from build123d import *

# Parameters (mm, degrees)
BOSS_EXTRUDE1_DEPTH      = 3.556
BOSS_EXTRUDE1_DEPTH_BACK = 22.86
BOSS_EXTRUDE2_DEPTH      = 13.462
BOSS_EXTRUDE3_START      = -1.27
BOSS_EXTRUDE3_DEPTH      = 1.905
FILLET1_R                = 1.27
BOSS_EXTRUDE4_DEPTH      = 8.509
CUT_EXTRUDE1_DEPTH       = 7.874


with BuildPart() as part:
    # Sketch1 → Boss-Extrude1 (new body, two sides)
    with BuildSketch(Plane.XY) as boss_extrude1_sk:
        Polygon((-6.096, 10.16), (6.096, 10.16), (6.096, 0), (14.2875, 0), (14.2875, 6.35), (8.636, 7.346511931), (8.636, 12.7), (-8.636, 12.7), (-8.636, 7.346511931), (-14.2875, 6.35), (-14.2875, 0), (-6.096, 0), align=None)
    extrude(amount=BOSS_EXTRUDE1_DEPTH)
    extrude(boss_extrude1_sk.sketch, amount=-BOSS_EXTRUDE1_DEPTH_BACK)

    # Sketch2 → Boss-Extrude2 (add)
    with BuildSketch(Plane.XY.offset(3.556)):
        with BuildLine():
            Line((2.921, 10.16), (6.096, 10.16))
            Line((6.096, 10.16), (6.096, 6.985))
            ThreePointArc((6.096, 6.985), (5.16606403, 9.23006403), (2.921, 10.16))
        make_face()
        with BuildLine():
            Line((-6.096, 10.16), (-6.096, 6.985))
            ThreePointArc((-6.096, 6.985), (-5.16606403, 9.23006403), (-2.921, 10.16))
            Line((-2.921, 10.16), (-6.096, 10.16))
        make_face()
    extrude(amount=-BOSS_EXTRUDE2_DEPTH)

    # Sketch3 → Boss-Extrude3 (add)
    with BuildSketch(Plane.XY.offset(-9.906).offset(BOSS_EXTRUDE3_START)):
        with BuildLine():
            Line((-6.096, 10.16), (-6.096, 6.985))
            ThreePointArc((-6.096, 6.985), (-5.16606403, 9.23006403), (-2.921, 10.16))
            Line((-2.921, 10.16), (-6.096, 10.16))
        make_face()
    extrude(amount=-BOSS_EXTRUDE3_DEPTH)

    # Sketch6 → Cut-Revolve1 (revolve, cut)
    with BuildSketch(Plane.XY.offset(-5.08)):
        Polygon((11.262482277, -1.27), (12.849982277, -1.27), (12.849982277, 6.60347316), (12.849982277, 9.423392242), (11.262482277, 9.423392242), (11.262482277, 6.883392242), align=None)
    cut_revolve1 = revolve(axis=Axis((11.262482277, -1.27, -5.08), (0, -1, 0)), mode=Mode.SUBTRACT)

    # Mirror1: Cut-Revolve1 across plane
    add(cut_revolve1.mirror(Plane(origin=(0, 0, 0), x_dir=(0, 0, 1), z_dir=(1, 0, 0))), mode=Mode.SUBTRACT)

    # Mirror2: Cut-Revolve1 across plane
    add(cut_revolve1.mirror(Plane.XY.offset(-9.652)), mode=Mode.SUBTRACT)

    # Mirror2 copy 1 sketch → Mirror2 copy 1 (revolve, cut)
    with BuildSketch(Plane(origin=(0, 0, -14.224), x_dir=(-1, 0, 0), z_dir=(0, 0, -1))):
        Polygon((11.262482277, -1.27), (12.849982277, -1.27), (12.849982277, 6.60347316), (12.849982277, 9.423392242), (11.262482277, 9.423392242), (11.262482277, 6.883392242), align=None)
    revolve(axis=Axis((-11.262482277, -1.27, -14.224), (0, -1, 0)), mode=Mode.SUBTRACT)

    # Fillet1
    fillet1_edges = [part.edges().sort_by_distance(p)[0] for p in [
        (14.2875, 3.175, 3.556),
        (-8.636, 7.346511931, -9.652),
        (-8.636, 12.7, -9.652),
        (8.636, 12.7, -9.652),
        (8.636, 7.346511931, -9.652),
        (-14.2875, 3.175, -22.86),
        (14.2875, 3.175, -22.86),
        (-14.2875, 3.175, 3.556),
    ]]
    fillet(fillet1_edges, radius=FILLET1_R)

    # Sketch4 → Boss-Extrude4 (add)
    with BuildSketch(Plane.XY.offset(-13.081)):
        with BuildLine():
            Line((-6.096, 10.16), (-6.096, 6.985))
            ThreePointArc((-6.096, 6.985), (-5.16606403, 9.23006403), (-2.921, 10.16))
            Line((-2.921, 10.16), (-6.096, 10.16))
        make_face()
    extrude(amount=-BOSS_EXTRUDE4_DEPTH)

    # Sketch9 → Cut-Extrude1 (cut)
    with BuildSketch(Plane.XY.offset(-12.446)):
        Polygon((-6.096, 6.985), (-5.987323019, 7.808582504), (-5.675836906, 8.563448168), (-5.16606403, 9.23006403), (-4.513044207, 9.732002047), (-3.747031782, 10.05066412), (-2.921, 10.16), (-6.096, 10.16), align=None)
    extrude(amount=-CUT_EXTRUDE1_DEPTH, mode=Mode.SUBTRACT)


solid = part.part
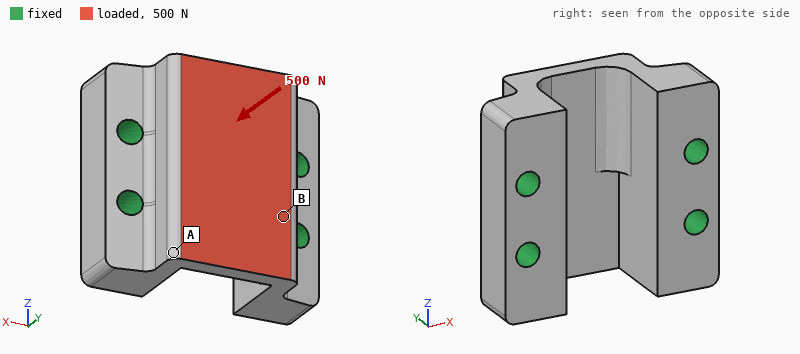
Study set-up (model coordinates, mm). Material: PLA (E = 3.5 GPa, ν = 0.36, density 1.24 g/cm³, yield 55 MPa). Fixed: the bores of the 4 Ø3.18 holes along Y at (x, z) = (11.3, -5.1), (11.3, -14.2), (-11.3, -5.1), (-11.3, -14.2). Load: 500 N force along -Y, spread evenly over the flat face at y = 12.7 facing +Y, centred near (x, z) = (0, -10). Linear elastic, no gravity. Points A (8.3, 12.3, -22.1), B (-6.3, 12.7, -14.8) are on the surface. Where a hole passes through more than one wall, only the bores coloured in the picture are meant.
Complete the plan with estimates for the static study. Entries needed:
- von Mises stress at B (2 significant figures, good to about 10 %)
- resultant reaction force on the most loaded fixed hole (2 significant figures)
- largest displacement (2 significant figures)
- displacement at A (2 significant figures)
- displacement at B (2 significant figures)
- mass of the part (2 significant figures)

4.2 MPa
160 N
66 µm
11 µm
19 µm
5.5 g
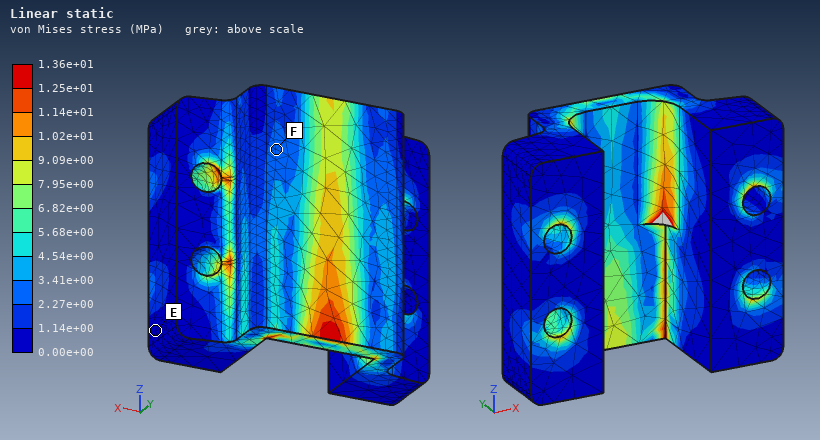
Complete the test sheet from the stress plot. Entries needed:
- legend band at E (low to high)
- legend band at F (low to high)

0.00e+00 to 1.14e+00 MPa
2.27e+00 to 3.41e+00 MPa
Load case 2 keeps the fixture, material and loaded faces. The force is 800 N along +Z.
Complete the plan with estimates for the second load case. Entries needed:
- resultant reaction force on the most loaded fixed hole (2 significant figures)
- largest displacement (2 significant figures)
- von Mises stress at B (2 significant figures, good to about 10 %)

310 N
0.12 mm
9.1 MPa
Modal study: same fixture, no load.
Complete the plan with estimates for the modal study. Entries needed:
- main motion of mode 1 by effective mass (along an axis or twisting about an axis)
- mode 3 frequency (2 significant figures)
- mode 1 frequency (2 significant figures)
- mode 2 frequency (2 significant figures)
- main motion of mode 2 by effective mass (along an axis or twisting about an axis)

along Z
14 kHz
12 kHz
12 kHz
along X
